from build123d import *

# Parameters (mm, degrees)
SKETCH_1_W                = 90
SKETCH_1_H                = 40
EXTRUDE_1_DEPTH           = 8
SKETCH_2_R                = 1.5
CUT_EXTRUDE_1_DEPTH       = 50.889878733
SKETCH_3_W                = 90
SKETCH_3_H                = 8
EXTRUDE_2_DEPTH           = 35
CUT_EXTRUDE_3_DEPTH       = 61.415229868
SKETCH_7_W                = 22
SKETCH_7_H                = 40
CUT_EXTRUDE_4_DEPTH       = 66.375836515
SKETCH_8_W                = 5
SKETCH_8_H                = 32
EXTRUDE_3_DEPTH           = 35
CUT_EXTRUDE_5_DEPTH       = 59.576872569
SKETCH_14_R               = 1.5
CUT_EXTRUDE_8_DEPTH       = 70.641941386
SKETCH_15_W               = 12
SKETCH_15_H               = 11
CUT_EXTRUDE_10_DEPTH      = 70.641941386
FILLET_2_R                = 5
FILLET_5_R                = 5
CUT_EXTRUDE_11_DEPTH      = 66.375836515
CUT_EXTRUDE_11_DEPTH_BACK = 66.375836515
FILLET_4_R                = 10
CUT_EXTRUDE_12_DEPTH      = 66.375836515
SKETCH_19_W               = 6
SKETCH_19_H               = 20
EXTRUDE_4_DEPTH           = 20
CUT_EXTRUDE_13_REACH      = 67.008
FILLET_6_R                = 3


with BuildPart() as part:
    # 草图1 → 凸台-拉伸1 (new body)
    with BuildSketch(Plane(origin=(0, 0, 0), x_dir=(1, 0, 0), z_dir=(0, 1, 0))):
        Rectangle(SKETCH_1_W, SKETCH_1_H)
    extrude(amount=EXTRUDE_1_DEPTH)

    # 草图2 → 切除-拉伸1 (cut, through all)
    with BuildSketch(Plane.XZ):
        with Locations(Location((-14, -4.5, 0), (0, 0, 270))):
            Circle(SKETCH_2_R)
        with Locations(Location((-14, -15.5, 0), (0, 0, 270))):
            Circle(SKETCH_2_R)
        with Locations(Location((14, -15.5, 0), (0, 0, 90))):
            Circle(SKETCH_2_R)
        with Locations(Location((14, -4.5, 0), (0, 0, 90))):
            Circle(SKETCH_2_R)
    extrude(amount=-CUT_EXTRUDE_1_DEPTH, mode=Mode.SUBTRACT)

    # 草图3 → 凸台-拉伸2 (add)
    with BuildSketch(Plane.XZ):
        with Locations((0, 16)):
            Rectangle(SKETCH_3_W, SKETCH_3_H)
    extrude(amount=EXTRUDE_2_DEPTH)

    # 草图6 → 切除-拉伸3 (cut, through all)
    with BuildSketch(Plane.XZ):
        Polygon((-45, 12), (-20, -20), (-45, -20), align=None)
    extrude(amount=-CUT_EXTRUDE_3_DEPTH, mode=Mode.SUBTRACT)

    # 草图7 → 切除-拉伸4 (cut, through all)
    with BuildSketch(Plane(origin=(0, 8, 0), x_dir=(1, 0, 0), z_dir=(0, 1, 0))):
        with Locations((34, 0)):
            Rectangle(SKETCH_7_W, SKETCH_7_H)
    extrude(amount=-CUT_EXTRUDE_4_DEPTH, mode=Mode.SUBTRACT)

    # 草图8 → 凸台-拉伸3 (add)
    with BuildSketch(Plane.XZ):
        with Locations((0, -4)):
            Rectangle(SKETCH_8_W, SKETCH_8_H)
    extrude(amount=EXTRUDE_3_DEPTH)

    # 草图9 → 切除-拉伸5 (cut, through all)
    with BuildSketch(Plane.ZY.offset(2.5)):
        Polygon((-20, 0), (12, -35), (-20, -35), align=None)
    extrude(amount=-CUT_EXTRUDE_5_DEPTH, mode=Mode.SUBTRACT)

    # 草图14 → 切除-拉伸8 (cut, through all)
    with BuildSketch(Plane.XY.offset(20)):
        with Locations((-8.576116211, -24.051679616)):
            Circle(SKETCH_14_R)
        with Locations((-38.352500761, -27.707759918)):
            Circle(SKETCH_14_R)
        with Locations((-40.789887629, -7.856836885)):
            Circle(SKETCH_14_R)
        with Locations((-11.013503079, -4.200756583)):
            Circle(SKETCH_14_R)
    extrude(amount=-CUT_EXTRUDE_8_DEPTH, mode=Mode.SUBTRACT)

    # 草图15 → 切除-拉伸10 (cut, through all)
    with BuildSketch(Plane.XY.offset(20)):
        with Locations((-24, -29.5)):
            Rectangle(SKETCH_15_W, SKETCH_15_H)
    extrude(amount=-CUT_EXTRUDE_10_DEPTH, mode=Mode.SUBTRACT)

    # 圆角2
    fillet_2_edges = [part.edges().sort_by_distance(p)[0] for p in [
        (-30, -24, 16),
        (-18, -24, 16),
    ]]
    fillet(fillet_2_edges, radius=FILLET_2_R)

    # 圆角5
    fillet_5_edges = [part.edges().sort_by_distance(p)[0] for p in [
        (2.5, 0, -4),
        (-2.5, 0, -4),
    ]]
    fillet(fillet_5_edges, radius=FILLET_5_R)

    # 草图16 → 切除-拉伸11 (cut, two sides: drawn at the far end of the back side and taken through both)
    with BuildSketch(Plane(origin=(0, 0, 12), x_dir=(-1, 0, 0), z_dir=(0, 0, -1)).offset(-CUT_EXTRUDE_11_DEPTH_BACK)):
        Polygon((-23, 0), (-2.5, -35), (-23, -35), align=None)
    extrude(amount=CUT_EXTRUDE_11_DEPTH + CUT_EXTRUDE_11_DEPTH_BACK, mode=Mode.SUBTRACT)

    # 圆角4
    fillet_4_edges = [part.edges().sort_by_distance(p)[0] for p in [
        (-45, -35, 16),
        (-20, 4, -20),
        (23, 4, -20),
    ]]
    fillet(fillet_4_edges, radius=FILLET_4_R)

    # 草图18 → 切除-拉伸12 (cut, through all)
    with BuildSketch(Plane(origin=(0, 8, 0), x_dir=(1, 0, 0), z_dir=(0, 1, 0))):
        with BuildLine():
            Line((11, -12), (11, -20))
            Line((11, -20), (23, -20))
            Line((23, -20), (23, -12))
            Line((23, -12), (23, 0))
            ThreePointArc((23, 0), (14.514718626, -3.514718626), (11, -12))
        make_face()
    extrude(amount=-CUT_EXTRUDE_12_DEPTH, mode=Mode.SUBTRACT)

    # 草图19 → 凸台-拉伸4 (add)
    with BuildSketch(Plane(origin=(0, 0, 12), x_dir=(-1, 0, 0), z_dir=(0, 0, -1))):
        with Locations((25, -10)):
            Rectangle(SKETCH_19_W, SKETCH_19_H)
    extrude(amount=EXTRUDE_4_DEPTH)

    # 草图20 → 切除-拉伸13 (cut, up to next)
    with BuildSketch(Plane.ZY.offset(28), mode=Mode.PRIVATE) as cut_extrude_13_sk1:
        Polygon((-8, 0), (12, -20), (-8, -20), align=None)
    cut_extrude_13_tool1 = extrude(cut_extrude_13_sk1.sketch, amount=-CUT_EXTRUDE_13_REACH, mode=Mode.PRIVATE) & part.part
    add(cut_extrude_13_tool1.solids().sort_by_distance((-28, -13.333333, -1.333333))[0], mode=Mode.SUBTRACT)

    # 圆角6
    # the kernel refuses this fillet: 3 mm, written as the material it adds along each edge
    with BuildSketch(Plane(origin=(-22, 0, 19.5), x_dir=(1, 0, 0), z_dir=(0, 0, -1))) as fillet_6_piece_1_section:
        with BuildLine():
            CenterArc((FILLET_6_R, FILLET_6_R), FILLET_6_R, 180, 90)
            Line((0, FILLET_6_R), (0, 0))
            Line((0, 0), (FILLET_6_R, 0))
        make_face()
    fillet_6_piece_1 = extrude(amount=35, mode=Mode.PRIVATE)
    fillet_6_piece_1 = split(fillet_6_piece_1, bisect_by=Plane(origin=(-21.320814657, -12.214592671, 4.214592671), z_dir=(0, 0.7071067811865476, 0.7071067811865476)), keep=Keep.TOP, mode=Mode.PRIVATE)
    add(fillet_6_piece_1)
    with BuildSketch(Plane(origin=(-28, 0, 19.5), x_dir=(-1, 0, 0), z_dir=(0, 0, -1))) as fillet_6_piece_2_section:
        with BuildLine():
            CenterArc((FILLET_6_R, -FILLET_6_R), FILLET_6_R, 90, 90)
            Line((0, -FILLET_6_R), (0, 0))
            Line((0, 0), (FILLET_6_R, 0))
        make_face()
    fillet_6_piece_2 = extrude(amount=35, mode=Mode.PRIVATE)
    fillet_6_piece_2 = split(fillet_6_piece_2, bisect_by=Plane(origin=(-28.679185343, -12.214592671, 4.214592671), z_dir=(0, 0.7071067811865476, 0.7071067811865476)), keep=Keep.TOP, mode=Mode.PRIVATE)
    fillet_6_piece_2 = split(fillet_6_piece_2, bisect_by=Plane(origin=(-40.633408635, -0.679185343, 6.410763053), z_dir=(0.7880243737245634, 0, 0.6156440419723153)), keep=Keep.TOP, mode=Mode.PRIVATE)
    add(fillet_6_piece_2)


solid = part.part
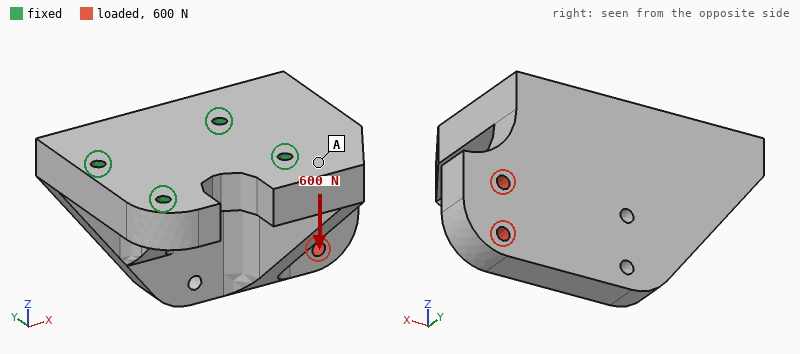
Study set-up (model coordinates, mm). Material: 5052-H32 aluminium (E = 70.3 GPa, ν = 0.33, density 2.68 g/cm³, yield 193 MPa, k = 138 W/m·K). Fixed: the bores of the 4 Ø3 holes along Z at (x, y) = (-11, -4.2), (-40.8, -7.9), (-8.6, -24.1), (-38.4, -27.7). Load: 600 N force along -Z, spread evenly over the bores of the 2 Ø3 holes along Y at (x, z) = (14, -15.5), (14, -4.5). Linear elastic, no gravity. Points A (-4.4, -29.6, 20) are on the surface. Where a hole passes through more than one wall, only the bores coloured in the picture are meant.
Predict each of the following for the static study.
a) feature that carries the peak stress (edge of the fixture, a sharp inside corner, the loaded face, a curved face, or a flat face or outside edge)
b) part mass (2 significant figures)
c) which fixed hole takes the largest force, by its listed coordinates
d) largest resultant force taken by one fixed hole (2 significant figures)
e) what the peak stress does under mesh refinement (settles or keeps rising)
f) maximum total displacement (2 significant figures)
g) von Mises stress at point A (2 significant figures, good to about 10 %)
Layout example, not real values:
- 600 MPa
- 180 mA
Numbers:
- edge of the fixture
- 93 g
- (-11, -4.2)
- 1.0 kN
- keeps rising
- 24 µm
- 3.6 MPa
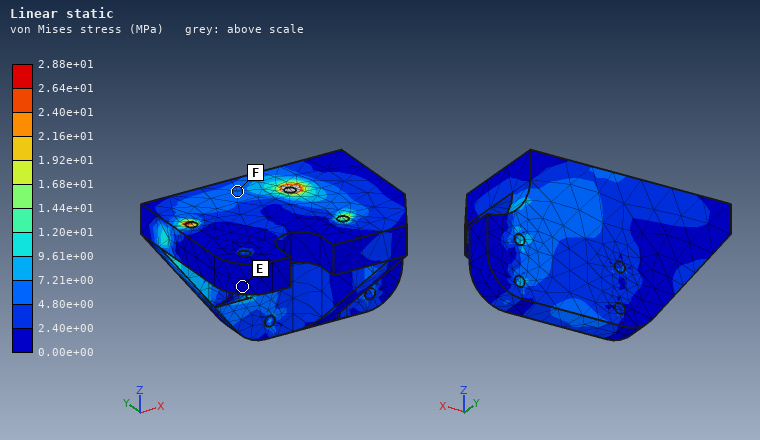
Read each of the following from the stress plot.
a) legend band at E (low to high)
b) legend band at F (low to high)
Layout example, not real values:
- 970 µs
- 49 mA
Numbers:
- 0.00e+00 to 2.40e+00 MPa
- 4.80e+00 to 7.21e+00 MPa
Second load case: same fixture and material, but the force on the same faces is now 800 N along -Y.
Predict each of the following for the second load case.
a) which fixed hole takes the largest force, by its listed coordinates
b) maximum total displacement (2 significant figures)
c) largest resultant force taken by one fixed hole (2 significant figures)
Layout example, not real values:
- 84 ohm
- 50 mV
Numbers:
- (-8.6, -24.1)
- 57 µm
- 1.2 kN
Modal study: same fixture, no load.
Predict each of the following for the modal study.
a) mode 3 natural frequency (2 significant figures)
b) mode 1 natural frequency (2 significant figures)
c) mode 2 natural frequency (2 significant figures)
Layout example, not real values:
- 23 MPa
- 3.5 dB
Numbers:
- 10 kHz
- 5600 Hz
- 7900 Hz
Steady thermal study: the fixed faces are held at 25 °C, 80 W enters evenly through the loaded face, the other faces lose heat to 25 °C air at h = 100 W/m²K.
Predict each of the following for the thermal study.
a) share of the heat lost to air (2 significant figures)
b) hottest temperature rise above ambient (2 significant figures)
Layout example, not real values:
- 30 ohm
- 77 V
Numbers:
- 23 %
- 77 K
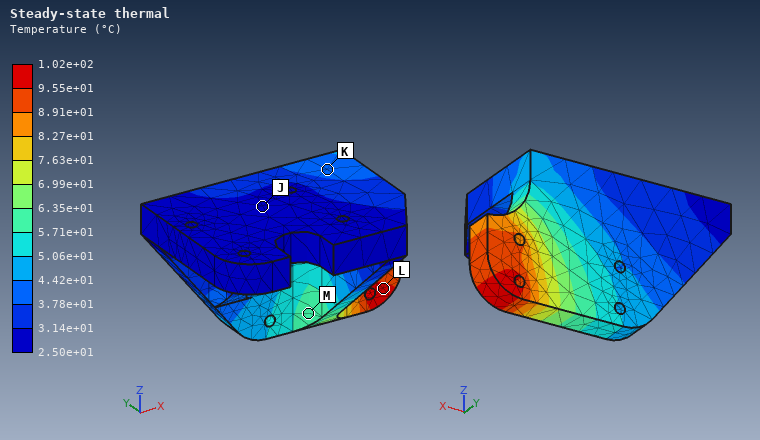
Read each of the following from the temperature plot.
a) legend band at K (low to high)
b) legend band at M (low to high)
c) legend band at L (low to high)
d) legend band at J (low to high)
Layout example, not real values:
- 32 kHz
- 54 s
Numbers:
- 3.78e+01 to 4.42e+01 °C
- 5.71e+01 to 6.35e+01 °C
- 9.55e+01 to 1.02e+02 °C
- 2.50e+01 to 3.14e+01 °C
